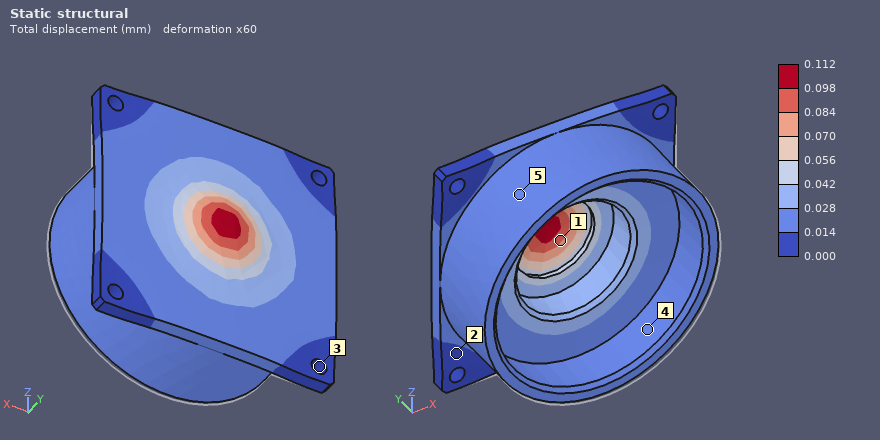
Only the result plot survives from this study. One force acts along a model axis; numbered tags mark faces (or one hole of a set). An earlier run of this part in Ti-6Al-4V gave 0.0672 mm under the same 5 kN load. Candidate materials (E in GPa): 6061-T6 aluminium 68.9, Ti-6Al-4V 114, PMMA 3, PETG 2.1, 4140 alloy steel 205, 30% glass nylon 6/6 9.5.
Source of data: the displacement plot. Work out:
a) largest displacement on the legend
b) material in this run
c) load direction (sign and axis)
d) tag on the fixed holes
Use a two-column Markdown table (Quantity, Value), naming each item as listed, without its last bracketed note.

| Quantity | Value |
|---|---|
| largest displacement on the legend | 0.112 mm |
| material in this run | 6061-T6 aluminium |
| load direction | +Y |
| tag on the fixed holes | 3 |
